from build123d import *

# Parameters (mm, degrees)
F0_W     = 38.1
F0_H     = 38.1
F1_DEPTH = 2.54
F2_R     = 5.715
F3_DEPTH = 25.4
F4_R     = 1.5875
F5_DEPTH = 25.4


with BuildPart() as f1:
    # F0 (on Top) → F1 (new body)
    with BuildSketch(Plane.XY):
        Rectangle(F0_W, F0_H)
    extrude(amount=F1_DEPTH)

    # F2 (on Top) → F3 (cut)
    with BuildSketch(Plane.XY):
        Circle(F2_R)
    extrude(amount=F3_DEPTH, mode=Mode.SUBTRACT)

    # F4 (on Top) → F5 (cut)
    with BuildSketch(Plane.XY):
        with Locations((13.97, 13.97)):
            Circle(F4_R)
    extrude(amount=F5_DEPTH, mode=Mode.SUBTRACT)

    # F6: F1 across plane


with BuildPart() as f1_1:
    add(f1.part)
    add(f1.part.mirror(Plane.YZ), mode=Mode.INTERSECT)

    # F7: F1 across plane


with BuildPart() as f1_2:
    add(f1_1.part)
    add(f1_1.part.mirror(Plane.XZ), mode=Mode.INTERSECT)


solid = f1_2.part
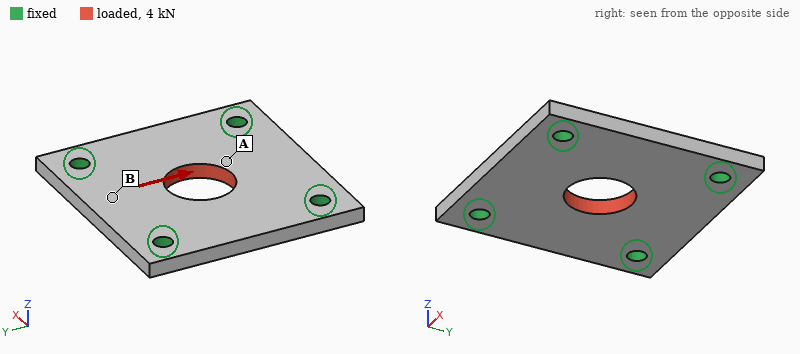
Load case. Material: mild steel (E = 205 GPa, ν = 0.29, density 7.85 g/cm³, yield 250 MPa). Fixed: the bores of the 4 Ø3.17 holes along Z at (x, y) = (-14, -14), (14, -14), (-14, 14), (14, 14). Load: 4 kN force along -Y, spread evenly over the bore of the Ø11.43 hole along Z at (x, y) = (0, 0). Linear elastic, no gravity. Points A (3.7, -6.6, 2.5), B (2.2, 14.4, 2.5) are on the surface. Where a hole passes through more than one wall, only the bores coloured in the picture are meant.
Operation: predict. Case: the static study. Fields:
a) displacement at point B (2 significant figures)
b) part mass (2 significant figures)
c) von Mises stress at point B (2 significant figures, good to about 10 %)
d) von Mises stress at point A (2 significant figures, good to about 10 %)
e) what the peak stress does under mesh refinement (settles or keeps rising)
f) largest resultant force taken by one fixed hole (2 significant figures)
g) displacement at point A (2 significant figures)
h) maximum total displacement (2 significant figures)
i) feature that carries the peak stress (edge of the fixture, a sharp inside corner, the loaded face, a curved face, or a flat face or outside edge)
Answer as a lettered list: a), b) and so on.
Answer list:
a) 3.3 µm
b) 26 g
c) 16 MPa
d) 39 MPa
e) keeps rising
f) 1.1 kN
g) 3.7 µm
h) 4.5 µm
i) edge of the fixture
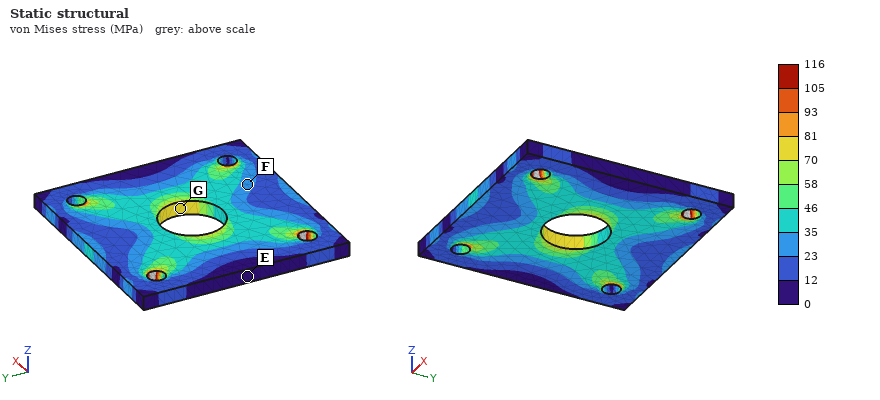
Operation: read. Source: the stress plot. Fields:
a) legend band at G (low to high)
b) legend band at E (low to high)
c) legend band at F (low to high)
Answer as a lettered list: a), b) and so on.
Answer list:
a) 70 to 81 MPa
b) 0 to 12 MPa
c) 23 to 35 MPa
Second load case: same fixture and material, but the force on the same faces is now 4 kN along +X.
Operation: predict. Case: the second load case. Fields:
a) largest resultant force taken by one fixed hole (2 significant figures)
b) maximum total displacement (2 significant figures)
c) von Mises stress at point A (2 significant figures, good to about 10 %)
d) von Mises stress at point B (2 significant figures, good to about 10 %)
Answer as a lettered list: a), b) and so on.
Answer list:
a) 1.1 kN
b) 4.5 µm
c) 50 MPa
d) 17 MPa
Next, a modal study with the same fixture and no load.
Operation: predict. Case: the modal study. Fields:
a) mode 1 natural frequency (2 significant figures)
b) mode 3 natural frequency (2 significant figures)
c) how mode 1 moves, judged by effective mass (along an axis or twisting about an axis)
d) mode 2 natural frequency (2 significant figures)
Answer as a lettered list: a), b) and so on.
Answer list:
a) 13 kHz
b) 19 kHz
c) along Z
d) 19 kHz
